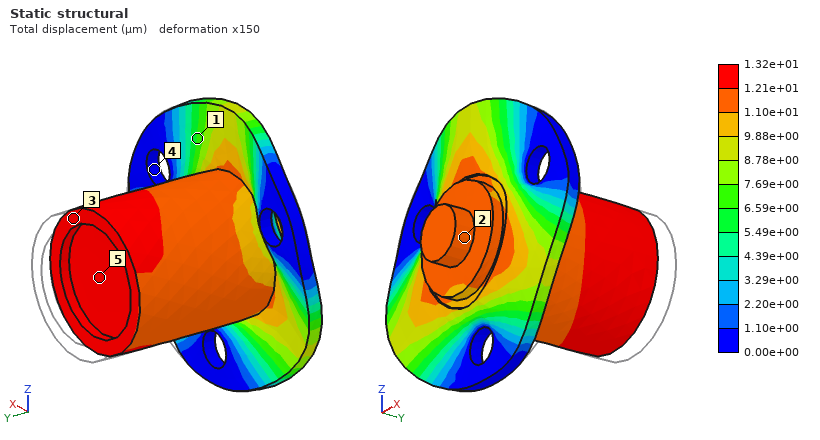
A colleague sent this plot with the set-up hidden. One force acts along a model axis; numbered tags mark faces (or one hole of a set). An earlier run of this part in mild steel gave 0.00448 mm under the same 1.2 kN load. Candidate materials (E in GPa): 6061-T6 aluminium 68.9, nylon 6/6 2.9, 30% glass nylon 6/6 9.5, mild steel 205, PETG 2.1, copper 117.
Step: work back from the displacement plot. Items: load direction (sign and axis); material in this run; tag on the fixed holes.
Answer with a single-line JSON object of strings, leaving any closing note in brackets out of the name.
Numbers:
{"load direction": "-Y", "material in this run": "6061-T6 aluminium", "tag on the fixed holes": "4"}
